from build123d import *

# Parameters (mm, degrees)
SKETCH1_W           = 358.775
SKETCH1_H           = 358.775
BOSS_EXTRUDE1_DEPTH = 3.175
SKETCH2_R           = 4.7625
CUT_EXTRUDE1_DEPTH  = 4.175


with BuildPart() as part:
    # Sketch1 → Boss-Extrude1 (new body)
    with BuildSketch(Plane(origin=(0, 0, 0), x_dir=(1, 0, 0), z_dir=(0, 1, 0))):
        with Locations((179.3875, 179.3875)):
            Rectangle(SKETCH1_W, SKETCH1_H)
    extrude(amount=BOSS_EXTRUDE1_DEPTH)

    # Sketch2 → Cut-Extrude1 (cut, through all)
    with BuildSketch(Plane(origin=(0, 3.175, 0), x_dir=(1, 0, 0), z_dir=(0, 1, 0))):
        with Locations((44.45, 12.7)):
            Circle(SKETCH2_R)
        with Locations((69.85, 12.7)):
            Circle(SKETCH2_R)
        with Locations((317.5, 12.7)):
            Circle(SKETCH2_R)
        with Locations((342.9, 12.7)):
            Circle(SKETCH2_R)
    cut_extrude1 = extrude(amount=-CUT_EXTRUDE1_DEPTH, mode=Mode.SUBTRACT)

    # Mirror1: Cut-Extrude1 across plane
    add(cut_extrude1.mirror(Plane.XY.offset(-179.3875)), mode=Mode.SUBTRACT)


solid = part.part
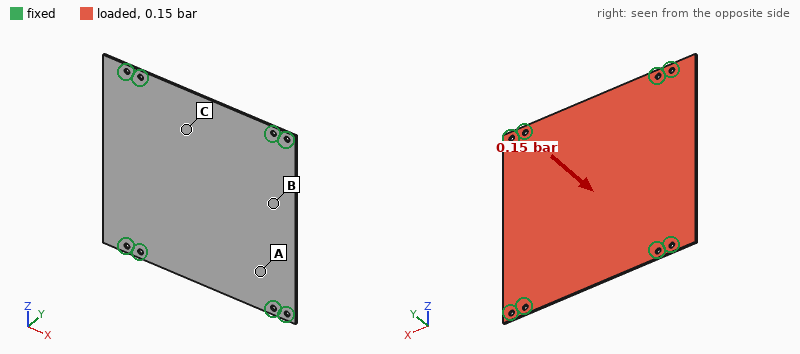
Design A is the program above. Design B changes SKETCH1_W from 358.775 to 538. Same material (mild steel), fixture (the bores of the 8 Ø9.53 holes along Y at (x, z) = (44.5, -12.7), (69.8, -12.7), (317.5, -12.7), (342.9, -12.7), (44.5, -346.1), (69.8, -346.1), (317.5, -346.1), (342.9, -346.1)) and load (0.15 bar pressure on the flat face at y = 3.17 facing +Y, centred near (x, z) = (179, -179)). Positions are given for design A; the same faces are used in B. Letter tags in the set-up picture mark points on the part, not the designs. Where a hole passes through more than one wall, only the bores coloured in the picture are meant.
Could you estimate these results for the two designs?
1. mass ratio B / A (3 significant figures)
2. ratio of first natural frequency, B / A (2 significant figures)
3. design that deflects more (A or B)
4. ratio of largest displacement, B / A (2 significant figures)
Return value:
1.50
0.74
B
2.1
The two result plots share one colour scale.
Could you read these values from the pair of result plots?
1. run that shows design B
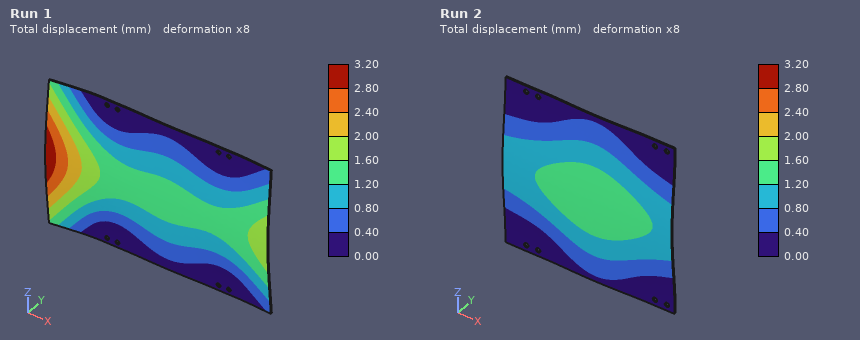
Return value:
Run 1
